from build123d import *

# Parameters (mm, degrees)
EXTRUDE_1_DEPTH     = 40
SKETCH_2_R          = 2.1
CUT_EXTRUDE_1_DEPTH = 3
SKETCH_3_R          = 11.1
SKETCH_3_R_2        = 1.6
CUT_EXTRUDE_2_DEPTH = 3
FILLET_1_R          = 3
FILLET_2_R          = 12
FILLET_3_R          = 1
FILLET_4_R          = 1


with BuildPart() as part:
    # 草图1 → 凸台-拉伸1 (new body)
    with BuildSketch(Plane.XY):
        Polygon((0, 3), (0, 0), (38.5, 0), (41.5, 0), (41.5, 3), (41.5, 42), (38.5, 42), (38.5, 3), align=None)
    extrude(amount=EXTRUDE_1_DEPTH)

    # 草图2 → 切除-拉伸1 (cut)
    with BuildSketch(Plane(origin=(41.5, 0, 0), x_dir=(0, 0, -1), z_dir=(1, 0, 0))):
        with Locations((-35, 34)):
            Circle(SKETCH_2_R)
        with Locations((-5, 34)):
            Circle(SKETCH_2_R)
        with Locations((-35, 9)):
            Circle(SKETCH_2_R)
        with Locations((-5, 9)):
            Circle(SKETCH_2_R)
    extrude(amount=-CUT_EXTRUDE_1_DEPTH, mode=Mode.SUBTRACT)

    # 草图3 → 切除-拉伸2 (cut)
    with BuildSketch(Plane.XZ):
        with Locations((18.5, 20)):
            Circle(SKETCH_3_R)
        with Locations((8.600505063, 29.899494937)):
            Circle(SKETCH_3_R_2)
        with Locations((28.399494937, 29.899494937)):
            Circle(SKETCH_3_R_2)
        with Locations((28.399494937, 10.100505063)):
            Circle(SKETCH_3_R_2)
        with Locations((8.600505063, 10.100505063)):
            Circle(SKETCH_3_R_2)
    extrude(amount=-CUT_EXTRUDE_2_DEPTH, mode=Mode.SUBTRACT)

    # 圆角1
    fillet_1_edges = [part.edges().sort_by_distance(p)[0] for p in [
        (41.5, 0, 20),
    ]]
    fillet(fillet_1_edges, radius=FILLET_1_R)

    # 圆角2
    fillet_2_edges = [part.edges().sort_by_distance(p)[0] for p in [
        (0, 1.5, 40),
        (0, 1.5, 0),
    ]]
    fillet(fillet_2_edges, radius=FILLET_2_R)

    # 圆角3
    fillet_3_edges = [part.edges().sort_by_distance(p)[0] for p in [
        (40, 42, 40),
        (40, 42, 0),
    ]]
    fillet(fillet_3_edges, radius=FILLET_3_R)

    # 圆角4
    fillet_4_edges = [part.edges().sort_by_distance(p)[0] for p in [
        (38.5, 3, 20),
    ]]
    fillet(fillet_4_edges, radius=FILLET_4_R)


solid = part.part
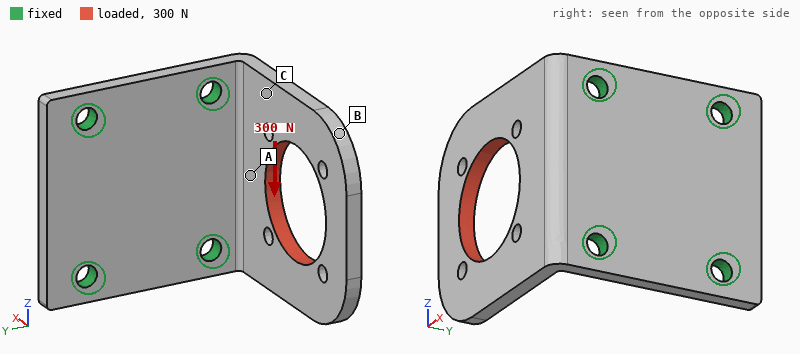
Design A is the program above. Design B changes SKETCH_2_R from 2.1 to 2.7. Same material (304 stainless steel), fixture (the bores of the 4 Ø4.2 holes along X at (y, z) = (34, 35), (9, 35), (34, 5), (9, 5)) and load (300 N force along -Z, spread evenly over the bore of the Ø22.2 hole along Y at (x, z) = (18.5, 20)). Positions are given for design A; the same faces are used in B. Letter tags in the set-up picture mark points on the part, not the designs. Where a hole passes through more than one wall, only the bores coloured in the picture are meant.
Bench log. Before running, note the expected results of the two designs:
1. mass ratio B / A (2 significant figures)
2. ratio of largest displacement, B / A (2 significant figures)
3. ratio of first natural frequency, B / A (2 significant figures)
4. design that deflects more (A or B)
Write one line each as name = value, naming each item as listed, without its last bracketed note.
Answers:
mass ratio B / A = 0.99
ratio of largest displacement, B / A = 0.86
ratio of first natural frequency, B / A = 1.0
design that deflects more = A
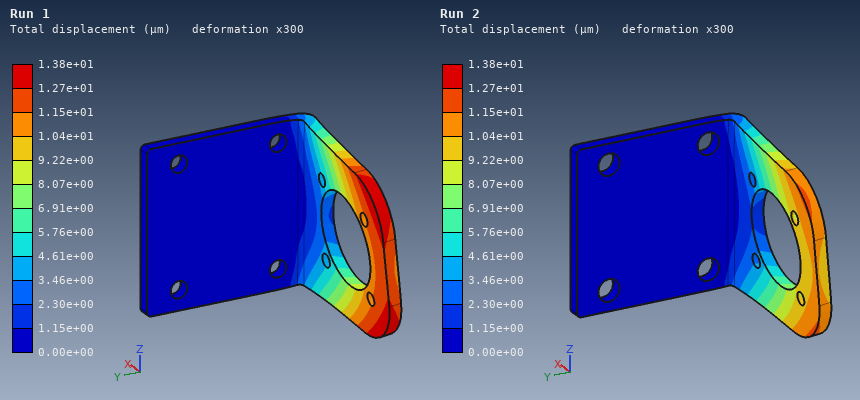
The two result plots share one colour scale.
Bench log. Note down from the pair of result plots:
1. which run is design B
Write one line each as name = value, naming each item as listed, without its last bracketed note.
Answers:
which run is design B = Run 2
